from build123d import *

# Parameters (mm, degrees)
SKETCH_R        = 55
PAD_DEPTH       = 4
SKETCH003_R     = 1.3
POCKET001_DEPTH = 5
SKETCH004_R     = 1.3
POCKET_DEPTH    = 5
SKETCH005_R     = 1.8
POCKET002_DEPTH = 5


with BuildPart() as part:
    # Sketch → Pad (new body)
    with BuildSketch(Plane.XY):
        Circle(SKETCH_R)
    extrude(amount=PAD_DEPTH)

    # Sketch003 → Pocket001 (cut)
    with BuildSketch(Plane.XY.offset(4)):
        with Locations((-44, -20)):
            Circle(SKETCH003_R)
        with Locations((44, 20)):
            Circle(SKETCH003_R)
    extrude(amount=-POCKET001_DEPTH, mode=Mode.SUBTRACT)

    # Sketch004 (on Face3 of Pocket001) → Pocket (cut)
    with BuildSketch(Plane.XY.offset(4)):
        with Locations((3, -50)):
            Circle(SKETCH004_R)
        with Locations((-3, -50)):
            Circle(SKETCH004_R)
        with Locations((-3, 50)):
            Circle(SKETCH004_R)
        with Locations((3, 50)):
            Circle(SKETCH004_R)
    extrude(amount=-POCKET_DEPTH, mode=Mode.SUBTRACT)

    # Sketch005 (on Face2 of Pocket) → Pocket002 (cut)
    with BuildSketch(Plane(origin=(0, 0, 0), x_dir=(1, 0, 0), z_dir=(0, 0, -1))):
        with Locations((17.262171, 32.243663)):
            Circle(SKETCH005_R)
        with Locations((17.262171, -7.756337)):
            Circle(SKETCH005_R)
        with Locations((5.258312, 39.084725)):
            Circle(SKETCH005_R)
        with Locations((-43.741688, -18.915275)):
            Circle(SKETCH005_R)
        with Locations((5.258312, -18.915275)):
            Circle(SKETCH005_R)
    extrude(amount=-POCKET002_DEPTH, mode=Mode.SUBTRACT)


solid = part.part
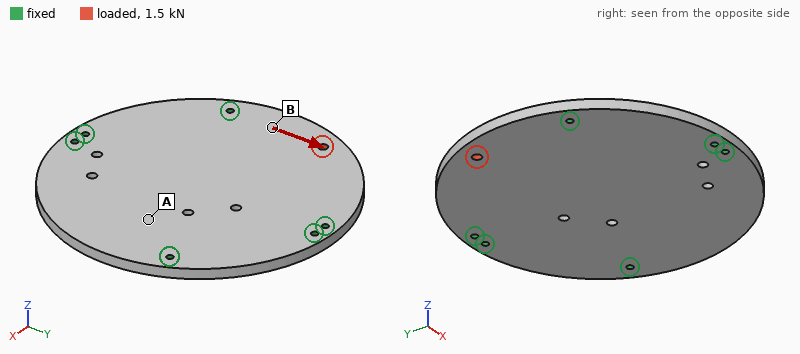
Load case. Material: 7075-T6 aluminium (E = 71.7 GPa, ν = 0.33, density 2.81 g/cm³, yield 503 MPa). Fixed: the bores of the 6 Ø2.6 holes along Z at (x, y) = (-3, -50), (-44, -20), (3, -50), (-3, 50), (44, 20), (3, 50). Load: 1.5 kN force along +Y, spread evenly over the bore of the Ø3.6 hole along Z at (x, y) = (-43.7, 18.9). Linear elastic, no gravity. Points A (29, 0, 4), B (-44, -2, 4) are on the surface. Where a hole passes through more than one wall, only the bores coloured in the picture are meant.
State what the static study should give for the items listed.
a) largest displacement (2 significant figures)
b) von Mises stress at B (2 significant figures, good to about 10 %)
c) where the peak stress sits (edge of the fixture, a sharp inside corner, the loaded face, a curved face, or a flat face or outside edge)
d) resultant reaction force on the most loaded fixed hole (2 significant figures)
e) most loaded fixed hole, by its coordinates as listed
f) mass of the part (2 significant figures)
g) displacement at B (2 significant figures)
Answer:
9.5 µm
12 MPa
the loaded face
850 N
(-44, -20)
110 g
3.7 µm
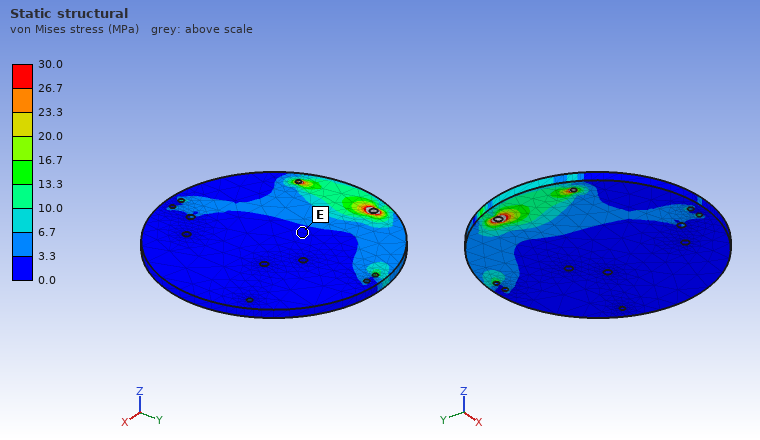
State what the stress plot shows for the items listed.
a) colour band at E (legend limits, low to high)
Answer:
0.0 to 3.3 MPa
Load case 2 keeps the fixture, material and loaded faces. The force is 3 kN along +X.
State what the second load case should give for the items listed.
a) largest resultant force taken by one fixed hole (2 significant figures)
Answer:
750 N
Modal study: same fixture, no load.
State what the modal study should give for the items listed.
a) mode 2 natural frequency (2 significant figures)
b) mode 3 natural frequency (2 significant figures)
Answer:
2300 Hz
3200 Hz
